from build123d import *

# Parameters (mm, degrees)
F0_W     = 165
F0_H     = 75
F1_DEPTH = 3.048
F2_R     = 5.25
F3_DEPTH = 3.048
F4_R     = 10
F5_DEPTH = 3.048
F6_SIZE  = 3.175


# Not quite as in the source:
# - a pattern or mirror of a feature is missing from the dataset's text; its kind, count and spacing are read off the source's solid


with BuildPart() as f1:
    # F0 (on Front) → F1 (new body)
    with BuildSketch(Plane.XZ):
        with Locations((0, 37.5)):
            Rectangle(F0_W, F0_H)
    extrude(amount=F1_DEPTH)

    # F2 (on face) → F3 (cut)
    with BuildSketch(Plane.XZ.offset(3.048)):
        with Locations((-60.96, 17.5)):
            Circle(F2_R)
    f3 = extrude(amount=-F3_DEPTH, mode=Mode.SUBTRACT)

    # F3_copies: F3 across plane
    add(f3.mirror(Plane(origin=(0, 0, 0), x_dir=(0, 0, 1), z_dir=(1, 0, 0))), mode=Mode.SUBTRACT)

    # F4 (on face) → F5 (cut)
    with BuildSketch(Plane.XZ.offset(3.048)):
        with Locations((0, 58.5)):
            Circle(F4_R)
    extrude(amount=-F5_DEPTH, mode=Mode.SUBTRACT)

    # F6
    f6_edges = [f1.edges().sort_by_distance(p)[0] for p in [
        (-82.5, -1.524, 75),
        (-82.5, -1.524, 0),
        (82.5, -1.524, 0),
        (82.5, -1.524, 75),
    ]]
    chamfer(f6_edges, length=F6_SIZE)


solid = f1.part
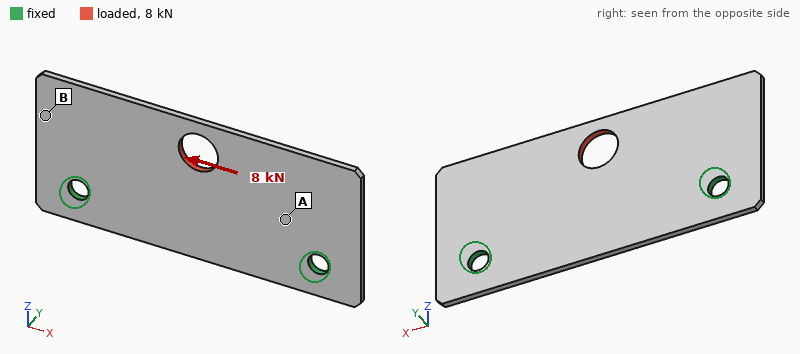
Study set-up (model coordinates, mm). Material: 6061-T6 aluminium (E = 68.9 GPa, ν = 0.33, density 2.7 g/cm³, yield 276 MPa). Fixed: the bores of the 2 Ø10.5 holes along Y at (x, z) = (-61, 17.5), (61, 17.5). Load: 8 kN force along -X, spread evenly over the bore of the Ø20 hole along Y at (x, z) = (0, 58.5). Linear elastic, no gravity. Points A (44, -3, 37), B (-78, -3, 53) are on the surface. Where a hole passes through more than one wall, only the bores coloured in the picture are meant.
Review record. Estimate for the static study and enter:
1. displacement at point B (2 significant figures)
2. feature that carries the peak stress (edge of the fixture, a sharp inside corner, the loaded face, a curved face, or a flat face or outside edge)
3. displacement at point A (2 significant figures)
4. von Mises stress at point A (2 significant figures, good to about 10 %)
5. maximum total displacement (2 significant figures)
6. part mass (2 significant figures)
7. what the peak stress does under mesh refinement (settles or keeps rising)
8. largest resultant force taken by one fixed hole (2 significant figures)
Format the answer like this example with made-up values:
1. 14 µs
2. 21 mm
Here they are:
1. 35 µm
2. edge of the fixture
3. 20 µm
4. 37 MPa
5. 64 µm
6. 98 g
7. keeps rising
8. 4.7 kN
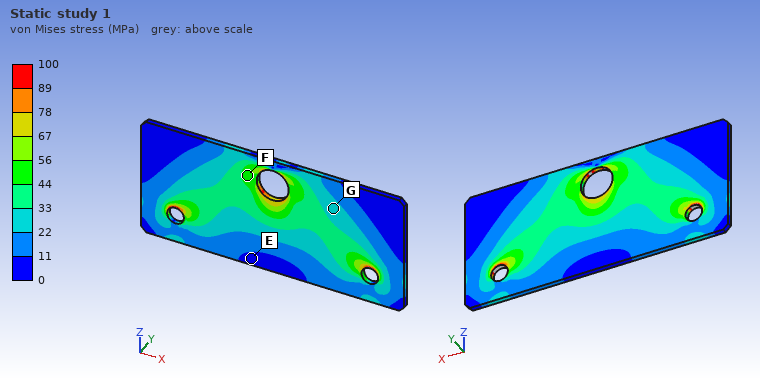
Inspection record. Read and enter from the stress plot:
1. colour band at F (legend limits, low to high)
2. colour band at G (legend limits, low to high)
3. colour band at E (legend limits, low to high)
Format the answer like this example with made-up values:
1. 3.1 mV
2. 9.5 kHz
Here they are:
1. 44 to 56 MPa
2. 22 to 33 MPa
3. 0 to 11 MPa
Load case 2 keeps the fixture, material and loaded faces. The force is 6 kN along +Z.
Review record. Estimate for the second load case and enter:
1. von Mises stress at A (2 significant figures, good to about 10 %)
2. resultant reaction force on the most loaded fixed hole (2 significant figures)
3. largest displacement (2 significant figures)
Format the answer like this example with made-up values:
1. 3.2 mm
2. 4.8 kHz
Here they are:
1. 35 MPa
2. 3.5 kN
3. 75 µm
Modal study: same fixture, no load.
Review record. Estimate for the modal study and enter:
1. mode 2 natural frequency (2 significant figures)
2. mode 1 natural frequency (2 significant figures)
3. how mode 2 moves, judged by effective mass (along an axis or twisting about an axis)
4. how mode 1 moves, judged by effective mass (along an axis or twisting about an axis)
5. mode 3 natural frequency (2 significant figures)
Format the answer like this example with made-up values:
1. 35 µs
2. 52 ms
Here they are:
1. 1000 Hz
2. 620 Hz
3. twisting about Z
4. along Y
5. 1100 Hz
